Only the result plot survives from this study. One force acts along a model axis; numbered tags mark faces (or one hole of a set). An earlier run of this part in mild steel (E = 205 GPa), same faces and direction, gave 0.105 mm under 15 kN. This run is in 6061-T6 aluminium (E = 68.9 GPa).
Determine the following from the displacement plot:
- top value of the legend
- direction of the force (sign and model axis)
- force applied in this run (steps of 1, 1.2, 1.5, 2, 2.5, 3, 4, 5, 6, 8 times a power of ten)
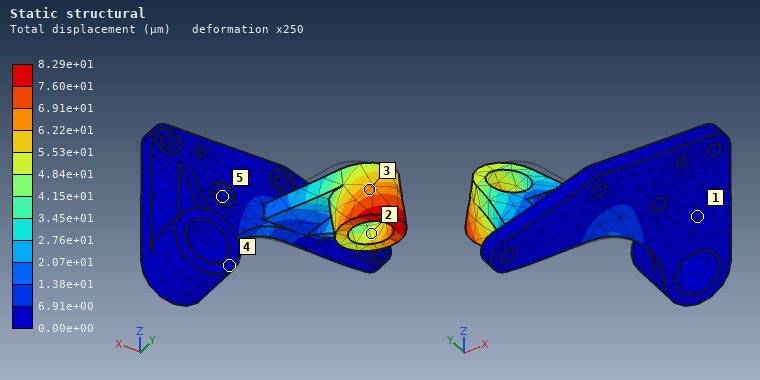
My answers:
8.29e+01 µm
-X
4 kN
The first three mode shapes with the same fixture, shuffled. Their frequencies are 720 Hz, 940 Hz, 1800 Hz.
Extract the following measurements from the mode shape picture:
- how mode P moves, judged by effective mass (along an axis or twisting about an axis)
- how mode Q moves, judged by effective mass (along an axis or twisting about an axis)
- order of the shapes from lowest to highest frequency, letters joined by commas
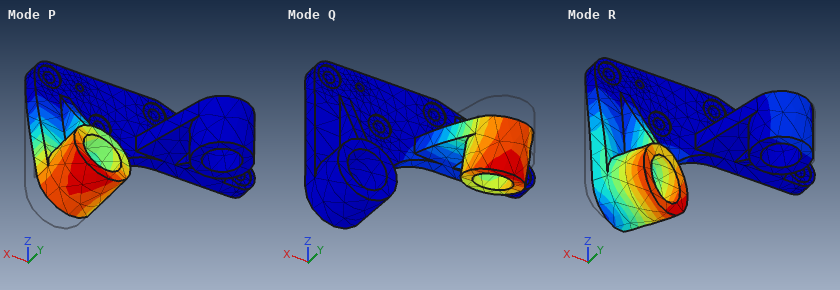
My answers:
along Y
along Z
P, Q, R
